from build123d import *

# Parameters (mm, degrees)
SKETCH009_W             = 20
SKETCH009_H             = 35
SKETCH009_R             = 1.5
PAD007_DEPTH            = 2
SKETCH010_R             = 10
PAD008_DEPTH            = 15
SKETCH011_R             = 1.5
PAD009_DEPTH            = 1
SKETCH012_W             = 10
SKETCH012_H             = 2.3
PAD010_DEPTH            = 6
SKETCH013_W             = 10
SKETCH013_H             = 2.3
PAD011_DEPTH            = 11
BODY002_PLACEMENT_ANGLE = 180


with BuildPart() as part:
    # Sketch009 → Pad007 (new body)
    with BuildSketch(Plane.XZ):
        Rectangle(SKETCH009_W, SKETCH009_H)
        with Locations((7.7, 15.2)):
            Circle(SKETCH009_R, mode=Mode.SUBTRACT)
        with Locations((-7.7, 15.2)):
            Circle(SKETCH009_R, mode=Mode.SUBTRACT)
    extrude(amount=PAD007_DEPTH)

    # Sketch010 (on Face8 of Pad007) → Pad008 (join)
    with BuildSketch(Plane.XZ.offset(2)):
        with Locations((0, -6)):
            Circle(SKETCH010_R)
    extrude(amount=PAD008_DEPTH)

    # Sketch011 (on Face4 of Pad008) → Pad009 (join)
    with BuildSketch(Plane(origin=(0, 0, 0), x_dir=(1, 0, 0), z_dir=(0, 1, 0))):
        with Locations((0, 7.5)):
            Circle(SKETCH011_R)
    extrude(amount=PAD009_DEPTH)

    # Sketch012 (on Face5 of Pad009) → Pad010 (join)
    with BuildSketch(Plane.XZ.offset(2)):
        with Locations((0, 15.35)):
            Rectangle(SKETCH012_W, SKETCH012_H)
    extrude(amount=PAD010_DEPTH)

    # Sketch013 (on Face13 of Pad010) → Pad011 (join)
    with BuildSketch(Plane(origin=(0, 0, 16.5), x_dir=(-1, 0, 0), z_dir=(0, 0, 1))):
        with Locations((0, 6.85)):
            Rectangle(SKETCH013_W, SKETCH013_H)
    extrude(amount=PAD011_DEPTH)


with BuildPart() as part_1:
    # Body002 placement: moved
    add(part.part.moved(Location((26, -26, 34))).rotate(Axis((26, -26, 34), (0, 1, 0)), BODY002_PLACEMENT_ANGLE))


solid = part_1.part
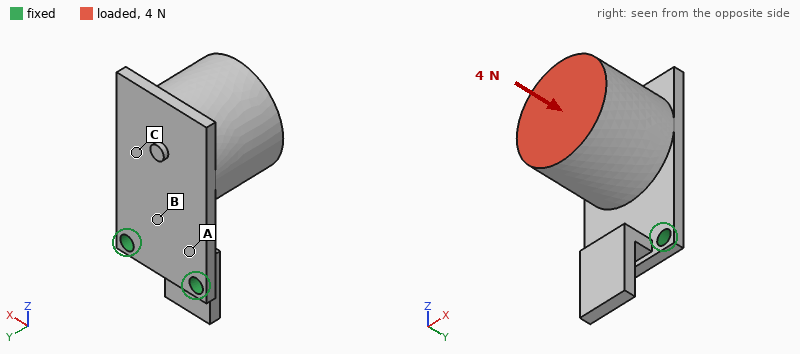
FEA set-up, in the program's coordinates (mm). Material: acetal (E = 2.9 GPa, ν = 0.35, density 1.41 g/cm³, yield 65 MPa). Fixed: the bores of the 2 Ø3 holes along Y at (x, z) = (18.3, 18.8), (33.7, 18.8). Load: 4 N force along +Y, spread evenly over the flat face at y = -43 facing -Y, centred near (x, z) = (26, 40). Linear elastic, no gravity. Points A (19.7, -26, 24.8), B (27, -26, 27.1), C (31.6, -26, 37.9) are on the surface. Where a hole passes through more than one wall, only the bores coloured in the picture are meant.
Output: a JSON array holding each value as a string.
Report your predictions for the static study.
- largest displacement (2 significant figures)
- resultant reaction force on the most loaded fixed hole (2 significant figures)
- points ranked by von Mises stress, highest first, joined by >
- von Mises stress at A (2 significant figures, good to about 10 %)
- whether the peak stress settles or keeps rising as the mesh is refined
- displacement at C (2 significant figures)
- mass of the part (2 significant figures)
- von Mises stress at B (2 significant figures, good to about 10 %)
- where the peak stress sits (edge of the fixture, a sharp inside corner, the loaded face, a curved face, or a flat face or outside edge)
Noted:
["0.54 mm", "2.0 N", "A > B > C", "4.4 MPa", "keeps rising", "0.25 mm", "9.1 g", "3.5 MPa", "edge of the fixture"]
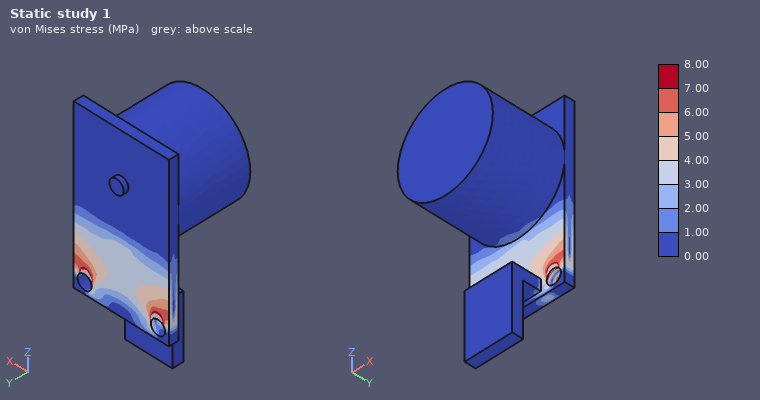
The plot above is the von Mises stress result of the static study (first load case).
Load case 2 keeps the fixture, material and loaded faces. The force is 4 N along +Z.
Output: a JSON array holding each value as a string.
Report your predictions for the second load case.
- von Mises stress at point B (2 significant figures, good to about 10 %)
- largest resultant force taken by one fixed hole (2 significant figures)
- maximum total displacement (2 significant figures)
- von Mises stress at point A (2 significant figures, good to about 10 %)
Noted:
["4.3 MPa", "2.3 N", "0.58 mm", "4.4 MPa"]
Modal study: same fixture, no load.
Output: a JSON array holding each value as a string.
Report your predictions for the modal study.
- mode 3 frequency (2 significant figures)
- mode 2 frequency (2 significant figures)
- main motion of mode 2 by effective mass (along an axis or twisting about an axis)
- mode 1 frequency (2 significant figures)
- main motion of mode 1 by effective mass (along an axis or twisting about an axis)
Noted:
["1400 Hz", "560 Hz", "along X", "180 Hz", "along Y"]
